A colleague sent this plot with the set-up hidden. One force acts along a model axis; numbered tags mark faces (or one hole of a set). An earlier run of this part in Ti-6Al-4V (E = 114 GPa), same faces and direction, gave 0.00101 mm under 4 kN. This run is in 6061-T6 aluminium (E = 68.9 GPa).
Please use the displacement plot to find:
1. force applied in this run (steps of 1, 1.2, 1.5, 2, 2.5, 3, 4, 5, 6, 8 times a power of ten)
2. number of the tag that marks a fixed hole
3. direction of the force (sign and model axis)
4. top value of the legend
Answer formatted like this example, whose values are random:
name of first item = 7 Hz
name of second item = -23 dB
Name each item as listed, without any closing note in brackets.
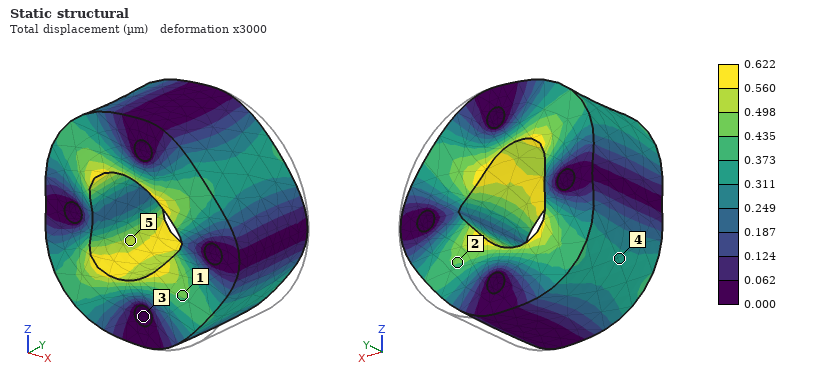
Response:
force applied in this run = 1.5 kN
number of the tag that marks a fixed hole = 3
direction of the force = -X
top value of the legend = 0.622 µm
